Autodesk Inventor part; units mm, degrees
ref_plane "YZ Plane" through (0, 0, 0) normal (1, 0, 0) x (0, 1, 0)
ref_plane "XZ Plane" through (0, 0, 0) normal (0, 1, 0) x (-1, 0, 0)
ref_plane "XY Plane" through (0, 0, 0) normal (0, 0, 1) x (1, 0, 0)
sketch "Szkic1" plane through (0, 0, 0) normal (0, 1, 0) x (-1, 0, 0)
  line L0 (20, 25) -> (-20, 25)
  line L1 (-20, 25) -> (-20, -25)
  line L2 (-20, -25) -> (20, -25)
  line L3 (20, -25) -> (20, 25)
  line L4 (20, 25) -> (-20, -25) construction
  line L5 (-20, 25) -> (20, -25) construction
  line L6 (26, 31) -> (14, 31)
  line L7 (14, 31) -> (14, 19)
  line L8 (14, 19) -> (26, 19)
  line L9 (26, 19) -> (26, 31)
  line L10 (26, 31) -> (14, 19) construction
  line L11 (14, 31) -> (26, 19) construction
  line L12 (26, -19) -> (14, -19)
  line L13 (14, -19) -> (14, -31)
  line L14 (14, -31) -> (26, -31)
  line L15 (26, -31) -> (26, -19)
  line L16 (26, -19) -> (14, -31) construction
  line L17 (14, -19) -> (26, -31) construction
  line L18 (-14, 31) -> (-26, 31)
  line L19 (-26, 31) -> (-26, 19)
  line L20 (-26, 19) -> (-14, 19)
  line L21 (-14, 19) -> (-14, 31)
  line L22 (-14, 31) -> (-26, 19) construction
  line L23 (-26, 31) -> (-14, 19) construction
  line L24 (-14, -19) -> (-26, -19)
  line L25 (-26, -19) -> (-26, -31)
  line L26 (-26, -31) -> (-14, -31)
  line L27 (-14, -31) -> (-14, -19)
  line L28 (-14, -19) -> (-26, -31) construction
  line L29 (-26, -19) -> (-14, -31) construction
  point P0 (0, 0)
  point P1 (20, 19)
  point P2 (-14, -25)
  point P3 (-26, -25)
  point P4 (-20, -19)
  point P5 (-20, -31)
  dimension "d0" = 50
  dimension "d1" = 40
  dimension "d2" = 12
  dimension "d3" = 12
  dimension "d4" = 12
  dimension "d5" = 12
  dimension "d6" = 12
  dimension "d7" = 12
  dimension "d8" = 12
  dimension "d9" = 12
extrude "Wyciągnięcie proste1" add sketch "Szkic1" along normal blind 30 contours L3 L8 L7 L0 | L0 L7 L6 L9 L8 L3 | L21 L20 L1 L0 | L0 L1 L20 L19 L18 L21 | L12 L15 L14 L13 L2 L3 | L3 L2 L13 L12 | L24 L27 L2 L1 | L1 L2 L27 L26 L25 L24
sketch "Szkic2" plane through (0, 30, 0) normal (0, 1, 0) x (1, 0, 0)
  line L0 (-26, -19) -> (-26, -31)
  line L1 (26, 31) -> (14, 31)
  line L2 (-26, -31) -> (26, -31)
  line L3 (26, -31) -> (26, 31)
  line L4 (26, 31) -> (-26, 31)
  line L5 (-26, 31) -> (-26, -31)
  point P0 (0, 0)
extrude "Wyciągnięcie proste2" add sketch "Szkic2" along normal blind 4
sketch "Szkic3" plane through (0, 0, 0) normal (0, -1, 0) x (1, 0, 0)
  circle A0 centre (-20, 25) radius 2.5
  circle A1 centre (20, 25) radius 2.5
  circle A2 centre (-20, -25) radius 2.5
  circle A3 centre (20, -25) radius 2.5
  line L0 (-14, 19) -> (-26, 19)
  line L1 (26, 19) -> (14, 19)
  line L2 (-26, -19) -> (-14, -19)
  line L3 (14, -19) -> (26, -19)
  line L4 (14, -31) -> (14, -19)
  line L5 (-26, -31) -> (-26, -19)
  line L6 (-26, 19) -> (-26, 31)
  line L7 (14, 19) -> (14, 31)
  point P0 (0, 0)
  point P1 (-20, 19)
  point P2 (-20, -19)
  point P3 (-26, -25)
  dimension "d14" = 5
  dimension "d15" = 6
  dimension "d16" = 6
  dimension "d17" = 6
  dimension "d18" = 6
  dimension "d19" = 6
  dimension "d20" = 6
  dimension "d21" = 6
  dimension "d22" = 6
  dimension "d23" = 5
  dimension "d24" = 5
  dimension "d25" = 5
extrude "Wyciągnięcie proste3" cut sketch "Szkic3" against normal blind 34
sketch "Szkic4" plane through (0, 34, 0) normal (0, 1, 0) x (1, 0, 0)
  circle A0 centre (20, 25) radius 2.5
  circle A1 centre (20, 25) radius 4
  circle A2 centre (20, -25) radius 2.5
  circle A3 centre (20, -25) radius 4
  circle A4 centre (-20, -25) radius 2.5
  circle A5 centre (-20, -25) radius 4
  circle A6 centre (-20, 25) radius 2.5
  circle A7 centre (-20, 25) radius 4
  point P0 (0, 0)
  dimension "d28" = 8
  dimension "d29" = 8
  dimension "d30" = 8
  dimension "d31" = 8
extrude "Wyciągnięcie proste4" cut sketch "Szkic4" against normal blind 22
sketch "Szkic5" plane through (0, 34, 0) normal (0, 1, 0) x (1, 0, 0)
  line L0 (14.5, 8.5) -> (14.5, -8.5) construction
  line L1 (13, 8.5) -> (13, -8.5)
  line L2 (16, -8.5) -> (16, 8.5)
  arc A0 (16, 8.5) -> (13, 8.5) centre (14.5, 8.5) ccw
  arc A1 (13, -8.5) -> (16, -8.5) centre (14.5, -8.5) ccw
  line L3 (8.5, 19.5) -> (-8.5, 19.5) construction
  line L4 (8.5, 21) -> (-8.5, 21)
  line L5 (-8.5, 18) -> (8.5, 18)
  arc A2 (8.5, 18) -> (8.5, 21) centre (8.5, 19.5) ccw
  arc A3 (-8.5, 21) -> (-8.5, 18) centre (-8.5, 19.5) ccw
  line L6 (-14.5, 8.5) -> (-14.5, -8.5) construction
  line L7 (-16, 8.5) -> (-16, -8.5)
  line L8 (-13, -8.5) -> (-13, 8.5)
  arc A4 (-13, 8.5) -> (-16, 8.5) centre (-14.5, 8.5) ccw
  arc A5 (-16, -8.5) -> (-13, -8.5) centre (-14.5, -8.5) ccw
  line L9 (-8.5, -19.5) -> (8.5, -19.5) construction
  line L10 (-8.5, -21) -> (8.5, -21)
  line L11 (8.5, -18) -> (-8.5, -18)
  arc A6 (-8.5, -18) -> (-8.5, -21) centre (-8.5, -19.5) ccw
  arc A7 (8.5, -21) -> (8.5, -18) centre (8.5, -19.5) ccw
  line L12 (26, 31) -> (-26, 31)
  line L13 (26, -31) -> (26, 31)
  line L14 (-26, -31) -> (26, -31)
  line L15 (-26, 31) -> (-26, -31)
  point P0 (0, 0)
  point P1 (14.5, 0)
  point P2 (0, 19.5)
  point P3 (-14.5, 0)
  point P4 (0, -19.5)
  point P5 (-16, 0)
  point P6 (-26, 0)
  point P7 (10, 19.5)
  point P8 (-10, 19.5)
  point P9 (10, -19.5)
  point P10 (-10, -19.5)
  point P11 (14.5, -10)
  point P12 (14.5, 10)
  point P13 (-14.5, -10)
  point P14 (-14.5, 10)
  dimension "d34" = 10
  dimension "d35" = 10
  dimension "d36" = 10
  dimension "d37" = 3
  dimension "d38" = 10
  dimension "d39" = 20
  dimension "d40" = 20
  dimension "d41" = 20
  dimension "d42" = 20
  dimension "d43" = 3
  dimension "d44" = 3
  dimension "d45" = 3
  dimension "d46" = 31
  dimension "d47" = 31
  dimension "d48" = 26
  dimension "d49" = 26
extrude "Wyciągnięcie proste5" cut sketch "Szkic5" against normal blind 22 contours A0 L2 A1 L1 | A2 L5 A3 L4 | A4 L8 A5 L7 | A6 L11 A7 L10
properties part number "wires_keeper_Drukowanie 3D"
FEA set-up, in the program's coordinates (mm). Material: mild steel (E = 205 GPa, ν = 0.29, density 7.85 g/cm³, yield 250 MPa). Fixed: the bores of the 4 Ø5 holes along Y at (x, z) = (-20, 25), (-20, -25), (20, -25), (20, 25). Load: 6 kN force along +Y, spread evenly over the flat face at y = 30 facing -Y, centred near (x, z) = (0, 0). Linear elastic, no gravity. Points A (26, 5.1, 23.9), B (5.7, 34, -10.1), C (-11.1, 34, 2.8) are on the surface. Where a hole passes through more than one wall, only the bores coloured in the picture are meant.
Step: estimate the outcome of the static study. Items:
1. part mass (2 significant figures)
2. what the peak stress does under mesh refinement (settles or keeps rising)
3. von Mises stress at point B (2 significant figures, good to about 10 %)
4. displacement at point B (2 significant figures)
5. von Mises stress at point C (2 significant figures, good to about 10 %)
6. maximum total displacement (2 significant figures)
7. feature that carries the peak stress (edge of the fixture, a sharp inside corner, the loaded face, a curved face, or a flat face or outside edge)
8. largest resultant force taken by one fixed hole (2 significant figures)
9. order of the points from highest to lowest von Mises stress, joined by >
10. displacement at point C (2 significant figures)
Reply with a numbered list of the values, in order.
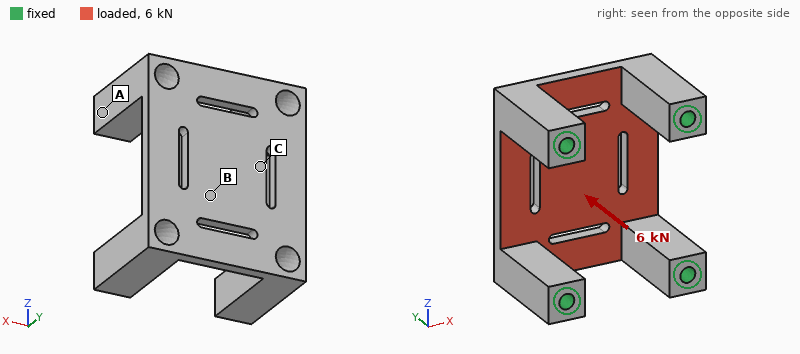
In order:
1. 190 g
2. keeps rising
3. 63 MPa
4. 37 µm
5. 100 MPa
6. 47 µm
7. a sharp inside corner
8. 1.6 kN
9. C > B > A
10. 43 µm
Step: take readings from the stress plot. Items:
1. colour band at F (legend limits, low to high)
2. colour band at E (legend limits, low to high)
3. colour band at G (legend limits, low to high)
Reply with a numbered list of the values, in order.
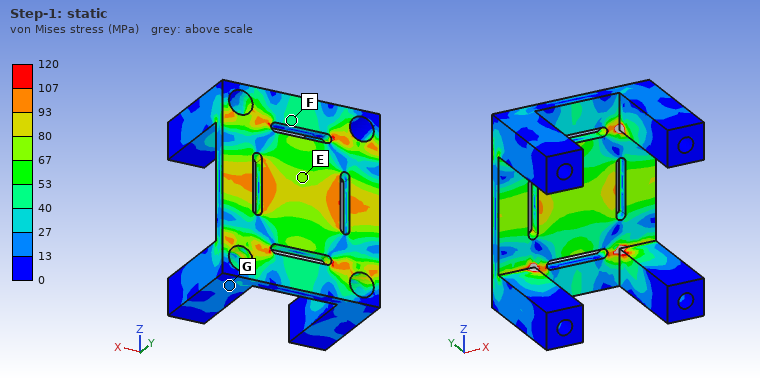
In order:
1. 40 to 53 MPa
2. 67 to 80 MPa
3. 13 to 27 MPa
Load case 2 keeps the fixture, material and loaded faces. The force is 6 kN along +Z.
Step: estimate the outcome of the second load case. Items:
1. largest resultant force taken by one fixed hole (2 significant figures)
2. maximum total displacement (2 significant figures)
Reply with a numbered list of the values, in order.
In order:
1. 1.5 kN
2. 35 µm
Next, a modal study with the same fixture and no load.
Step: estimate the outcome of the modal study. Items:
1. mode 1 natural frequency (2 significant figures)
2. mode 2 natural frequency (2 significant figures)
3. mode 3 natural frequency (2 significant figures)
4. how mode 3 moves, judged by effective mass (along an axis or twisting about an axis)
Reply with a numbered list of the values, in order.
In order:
1. 6800 Hz
2. 7000 Hz
3. 7800 Hz
4. along Y
